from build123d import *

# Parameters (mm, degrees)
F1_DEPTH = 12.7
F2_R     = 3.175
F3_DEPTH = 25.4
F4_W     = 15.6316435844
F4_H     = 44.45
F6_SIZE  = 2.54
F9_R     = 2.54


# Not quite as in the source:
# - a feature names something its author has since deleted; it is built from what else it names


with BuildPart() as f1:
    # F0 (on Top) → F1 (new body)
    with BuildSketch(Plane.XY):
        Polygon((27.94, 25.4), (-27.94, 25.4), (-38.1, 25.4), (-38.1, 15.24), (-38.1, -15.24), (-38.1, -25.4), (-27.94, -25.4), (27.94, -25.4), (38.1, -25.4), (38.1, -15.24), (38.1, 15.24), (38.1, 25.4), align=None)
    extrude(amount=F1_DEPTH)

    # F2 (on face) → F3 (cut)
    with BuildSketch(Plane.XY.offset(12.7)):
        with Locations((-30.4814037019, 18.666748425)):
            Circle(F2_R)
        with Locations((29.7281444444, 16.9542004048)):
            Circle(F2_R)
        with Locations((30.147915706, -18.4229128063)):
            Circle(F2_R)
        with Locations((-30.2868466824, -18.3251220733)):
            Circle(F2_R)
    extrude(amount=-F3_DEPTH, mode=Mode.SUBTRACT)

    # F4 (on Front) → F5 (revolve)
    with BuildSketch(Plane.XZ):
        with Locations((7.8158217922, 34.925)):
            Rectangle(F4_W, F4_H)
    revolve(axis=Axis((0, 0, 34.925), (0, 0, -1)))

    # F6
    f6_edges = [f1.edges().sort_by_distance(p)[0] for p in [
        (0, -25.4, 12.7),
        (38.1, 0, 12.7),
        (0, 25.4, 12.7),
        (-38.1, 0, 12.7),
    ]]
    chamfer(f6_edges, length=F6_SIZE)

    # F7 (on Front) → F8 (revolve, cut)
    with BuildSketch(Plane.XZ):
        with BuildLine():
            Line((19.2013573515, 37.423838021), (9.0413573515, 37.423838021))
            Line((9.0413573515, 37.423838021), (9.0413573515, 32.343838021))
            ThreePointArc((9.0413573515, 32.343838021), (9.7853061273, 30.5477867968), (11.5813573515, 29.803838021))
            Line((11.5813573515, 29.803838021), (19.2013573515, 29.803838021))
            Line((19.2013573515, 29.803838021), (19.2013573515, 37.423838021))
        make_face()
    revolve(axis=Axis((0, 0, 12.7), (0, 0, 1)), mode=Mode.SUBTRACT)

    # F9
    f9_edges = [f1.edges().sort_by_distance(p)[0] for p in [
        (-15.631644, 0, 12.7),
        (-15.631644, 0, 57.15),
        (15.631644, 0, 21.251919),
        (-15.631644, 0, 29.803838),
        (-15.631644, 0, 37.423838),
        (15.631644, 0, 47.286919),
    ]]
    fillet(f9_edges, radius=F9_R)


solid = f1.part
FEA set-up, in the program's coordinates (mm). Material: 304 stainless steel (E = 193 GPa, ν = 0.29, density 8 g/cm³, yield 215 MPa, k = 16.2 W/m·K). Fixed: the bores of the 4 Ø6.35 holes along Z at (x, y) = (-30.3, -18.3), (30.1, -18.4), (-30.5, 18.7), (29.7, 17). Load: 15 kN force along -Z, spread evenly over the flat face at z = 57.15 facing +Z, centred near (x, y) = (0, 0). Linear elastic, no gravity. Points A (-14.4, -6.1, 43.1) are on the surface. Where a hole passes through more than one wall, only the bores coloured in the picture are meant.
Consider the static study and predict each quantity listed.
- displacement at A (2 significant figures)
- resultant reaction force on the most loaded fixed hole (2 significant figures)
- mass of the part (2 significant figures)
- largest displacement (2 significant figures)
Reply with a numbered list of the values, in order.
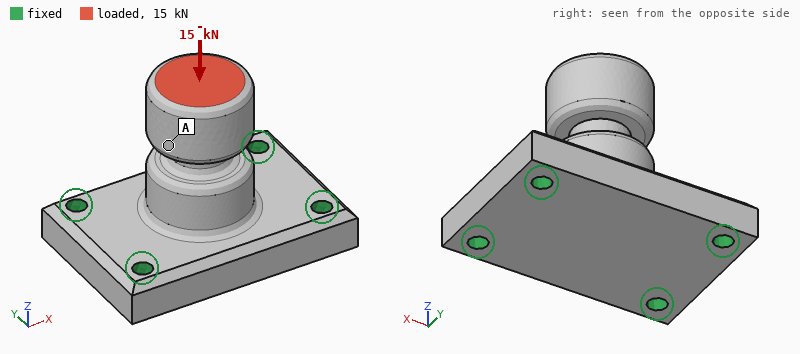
1. 17 µm
2. 4.1 kN
3. 610 g
4. 18 µm
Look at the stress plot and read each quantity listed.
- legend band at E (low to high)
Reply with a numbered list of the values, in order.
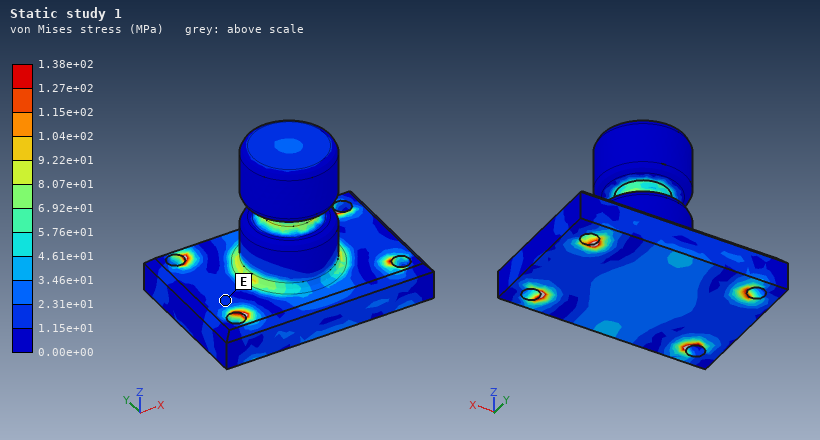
1. 1.15e+01 to 2.31e+01 MPa
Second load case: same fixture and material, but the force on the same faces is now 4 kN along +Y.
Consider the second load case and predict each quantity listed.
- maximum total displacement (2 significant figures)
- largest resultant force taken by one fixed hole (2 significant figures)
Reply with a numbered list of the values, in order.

1. 72 µm
2. 3.1 kN
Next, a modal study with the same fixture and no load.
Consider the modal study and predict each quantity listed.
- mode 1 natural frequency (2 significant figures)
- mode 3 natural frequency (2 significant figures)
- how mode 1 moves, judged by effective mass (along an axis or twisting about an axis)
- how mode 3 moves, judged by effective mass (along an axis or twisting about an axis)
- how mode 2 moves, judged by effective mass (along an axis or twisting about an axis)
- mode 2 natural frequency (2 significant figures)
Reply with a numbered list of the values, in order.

1. 4400 Hz
2. 9200 Hz
3. along Y
4. along Z
5. along X
6. 5100 Hz
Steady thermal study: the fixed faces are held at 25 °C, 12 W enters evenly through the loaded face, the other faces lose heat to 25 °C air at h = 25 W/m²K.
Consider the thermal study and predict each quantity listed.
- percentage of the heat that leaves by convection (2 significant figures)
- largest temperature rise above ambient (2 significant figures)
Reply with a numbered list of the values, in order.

1. 43 %
2. 63 K
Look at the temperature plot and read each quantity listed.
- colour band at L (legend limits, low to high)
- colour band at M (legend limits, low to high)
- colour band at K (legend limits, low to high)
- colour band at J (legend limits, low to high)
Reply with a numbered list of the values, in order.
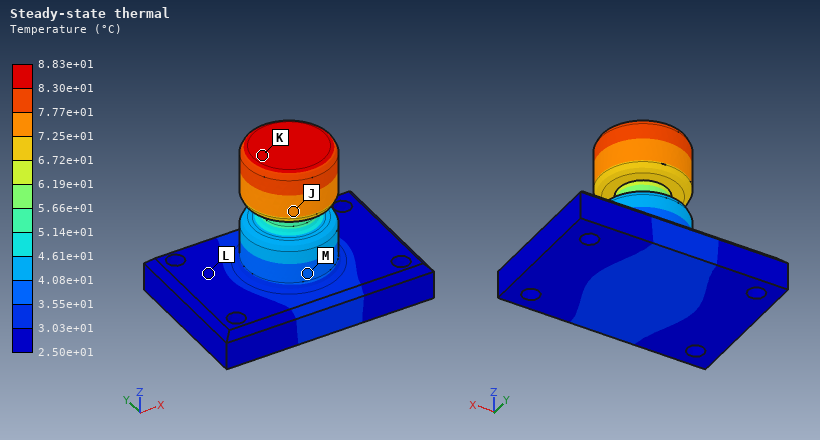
1. 2.50e+01 to 3.03e+01 °C
2. 3.55e+01 to 4.08e+01 °C
3. 8.30e+01 to 8.83e+01 °C
4. 7.25e+01 to 7.77e+01 °C
